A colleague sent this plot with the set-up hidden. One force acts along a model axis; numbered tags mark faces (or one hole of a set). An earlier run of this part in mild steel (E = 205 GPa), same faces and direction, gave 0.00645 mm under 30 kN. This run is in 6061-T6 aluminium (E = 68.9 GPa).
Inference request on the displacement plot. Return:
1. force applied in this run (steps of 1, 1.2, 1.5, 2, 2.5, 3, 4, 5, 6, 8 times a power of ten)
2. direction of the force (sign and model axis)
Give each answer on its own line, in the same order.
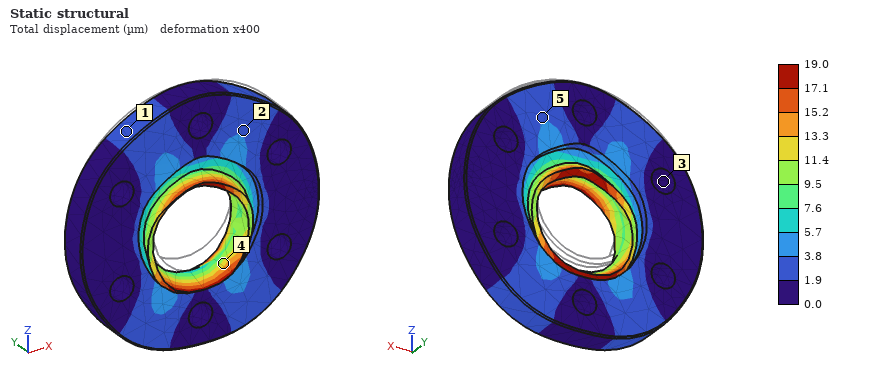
30 kN
-Z
